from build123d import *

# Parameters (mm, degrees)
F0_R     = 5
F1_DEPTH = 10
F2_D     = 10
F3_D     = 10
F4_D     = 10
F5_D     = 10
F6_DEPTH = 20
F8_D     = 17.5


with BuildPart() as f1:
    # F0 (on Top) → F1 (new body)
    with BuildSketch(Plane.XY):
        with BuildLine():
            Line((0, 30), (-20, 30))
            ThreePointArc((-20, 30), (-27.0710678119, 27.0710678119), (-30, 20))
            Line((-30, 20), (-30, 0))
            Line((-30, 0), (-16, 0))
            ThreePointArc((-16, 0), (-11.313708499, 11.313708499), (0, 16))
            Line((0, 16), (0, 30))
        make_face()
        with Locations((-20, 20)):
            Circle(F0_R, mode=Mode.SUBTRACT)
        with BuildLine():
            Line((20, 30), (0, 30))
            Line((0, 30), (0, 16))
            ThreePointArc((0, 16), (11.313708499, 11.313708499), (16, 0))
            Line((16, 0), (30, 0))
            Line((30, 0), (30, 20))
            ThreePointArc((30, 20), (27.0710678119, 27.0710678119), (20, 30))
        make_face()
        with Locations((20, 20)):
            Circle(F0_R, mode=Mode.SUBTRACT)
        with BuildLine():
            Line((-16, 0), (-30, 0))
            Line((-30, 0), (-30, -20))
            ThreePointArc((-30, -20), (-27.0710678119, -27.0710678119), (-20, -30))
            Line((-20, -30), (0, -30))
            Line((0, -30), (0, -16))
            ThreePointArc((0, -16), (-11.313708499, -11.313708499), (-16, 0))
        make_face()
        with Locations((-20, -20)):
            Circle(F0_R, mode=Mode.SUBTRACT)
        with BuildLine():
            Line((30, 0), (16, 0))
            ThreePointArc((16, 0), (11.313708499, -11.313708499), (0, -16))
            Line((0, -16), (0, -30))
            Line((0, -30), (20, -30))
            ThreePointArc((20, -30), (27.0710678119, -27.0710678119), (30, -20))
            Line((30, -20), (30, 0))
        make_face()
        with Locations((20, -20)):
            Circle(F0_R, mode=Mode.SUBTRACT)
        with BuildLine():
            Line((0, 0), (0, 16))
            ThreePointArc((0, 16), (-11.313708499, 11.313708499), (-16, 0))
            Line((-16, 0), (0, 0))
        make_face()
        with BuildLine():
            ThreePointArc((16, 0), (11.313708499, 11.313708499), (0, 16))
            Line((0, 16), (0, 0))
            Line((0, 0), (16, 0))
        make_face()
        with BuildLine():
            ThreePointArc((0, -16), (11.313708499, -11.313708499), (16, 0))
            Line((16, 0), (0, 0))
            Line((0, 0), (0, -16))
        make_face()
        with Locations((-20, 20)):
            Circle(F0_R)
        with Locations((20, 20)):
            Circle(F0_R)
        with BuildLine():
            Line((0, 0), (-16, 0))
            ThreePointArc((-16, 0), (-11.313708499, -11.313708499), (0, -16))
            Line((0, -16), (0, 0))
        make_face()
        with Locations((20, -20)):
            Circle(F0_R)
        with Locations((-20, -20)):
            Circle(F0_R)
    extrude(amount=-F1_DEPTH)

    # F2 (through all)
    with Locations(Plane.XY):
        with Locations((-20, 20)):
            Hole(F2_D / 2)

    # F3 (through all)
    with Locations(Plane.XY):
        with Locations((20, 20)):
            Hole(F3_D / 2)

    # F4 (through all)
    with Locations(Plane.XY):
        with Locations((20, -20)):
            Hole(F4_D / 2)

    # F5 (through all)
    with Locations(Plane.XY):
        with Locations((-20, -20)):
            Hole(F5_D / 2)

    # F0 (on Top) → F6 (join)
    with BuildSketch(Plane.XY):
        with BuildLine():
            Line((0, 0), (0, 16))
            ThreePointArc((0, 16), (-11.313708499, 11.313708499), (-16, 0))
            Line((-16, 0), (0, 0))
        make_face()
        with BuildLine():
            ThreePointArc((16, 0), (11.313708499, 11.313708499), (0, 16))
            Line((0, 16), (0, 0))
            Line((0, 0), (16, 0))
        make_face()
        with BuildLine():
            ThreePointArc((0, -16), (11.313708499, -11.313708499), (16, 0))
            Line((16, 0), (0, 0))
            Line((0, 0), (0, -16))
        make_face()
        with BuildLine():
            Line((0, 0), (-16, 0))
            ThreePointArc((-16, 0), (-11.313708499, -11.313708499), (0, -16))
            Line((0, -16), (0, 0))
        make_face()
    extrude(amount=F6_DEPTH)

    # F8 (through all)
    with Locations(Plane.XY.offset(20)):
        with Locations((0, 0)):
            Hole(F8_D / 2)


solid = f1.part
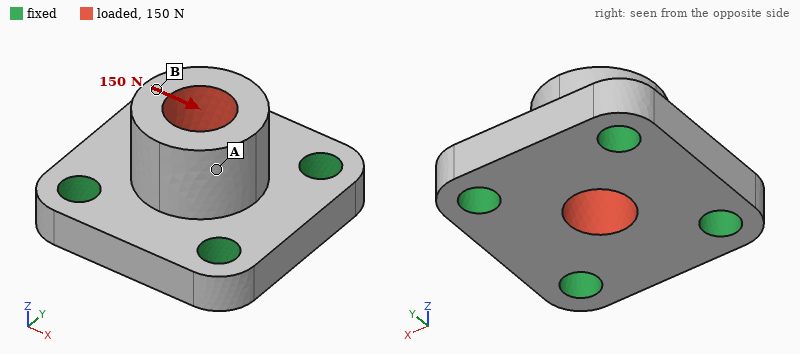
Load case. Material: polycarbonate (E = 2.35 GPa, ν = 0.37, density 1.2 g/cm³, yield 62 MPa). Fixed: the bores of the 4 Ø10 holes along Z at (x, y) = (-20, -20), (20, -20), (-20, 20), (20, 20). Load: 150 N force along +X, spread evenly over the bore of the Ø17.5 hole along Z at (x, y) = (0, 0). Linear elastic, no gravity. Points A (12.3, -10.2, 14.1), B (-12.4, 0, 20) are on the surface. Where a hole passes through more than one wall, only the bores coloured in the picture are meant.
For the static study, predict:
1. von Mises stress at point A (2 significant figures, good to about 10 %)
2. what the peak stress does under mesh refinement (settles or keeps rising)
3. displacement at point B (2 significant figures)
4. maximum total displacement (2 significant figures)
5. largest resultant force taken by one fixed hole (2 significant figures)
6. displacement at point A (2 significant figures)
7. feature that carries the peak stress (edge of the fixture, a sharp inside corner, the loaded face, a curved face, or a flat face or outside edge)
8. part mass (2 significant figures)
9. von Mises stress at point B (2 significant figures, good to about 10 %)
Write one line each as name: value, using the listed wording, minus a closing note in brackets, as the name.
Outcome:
von Mises stress at point A: 0.11 MPa
what the peak stress does under mesh refinement: keeps rising
displacement at point B: 10 µm
maximum total displacement: 11 µm
largest resultant force taken by one fixed hole: 46 N
displacement at point A: 8.2 µm
feature that carries the peak stress: edge of the fixture
part mass: 49 g
von Mises stress at point B: 0.23 MPa
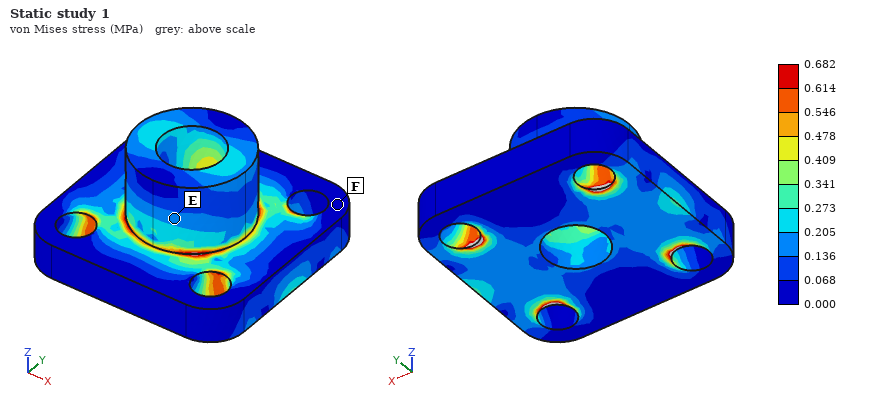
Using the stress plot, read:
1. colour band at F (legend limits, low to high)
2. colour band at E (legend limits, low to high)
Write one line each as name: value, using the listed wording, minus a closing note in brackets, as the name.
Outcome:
colour band at F: 0.000 to 0.068 MPa
colour band at E: 0.136 to 0.205 MPa
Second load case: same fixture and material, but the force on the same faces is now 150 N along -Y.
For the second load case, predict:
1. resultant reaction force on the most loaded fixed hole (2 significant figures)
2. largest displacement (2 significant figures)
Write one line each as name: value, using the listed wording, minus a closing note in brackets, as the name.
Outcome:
resultant reaction force on the most loaded fixed hole: 46 N
largest displacement: 11 µm
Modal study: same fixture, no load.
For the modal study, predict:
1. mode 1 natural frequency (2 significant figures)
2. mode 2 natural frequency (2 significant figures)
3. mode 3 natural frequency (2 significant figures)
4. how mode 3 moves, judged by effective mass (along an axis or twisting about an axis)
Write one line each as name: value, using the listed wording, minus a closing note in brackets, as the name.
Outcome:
mode 1 natural frequency: 4800 Hz
mode 2 natural frequency: 4800 Hz
mode 3 natural frequency: 5600 Hz
how mode 3 moves, judged by effective mass: along Z
